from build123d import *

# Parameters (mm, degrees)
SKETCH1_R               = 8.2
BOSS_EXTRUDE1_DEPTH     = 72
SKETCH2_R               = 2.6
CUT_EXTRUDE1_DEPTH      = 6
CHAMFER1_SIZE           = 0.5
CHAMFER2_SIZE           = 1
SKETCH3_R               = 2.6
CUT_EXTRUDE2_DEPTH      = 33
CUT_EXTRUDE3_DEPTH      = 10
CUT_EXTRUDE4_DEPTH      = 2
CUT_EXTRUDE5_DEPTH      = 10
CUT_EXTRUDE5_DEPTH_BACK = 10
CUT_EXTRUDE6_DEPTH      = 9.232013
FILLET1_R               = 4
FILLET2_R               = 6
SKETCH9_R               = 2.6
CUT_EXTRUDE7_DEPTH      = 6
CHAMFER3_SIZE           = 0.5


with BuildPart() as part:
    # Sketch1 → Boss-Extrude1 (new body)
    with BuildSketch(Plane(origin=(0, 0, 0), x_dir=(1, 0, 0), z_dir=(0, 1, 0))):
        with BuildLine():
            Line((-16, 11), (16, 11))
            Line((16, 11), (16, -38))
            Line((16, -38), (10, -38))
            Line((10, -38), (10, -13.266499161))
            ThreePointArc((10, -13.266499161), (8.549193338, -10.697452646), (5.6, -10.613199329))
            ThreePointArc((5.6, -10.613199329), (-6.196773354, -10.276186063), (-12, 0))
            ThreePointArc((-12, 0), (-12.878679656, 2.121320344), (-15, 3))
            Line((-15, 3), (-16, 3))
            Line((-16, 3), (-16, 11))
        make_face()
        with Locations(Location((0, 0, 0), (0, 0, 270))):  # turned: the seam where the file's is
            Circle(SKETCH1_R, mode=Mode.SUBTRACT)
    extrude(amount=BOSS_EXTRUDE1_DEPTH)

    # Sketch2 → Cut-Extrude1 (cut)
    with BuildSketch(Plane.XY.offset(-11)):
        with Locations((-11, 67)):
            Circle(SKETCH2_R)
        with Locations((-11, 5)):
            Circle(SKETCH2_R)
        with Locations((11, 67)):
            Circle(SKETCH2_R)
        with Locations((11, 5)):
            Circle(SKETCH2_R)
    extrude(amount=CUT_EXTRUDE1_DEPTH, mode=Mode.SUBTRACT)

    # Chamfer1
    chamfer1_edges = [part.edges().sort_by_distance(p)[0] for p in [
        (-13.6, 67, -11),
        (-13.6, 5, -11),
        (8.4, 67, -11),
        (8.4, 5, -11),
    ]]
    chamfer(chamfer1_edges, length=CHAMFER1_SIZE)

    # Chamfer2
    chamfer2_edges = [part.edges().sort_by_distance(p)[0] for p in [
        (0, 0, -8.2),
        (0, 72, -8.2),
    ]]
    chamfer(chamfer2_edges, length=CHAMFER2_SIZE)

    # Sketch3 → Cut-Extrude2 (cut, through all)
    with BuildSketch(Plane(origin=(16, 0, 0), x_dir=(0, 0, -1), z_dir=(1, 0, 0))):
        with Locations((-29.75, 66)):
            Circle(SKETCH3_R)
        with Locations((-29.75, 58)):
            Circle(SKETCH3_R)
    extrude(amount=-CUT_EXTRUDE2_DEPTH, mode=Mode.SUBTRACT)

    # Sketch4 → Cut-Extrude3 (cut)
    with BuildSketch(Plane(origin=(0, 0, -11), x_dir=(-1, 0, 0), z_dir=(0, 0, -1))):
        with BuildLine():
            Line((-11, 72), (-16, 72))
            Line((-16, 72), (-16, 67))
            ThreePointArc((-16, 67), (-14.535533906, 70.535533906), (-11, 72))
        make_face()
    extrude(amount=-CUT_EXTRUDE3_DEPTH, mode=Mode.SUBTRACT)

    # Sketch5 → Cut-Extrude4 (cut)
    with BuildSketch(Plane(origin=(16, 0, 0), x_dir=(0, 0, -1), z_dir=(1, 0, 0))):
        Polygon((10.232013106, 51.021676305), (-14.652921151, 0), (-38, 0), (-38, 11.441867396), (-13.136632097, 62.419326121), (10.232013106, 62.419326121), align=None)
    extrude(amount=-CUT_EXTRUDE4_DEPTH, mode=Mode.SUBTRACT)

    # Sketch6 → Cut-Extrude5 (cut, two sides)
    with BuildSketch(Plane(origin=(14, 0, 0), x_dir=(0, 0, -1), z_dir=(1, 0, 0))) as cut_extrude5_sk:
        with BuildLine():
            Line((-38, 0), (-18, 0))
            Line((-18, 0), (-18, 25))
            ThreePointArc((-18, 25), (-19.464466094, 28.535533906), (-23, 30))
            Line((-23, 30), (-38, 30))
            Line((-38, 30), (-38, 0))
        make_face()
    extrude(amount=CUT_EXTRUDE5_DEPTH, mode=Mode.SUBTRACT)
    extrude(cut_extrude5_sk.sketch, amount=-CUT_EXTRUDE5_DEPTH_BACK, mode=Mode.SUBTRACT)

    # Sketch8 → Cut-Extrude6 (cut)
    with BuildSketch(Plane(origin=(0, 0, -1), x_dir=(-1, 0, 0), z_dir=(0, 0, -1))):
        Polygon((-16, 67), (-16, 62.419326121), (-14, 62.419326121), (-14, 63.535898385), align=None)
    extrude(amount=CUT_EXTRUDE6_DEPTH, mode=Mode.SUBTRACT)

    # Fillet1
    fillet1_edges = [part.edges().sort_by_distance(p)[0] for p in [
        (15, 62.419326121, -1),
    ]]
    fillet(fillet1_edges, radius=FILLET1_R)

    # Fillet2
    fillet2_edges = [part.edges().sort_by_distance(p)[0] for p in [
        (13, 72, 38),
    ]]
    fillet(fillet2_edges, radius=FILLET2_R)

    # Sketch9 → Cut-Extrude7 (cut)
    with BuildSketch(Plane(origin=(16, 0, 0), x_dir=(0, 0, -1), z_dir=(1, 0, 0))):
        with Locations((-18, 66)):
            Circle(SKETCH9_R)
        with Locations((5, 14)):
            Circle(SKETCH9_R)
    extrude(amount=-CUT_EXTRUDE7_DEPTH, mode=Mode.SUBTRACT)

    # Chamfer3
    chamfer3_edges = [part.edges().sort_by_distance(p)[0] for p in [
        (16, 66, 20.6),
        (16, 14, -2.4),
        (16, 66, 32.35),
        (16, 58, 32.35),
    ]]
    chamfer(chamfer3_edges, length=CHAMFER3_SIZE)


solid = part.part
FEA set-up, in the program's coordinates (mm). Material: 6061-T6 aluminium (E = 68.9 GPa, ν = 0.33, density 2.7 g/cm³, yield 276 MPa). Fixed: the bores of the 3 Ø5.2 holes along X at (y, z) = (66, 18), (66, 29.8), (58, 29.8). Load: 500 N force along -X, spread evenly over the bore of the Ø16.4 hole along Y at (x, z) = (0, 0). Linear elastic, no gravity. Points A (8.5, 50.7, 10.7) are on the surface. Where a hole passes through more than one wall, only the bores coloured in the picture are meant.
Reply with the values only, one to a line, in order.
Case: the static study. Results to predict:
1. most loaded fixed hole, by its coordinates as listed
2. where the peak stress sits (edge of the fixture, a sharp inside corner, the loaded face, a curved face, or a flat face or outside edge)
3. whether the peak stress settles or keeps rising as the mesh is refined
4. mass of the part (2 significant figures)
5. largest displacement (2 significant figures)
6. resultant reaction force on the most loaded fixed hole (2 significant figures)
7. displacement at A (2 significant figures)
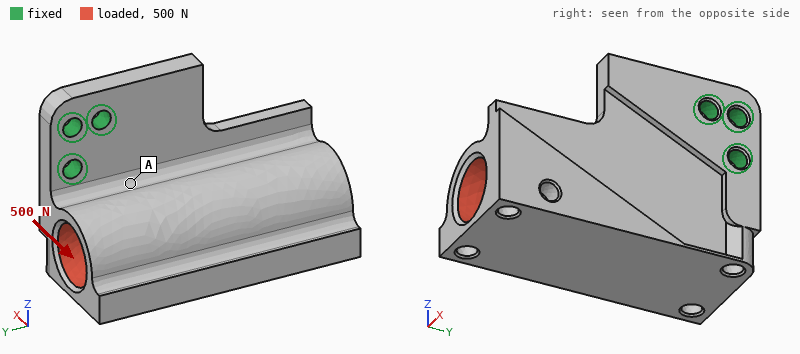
(66, 18)
edge of the fixture
keeps rising
94 g
0.30 mm
380 N
0.048 mm
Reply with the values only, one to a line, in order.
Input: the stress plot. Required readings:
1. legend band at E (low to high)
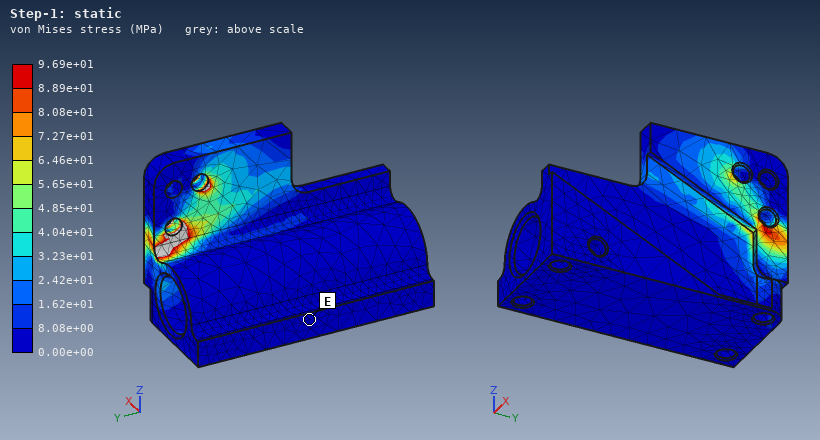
0.00e+00 to 8.08e+00 MPa
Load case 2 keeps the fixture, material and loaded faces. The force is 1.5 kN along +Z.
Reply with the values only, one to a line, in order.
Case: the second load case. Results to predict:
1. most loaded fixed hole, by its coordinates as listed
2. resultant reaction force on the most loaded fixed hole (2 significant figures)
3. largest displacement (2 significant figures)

(58, 29.8)
2.4 kN
0.38 mm
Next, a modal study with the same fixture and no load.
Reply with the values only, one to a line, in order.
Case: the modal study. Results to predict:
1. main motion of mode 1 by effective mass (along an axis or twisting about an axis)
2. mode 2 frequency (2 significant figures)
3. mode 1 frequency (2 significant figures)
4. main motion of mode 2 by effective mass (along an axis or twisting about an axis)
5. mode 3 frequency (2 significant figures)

along X
2000 Hz
890 Hz
along Z
3400 Hz
